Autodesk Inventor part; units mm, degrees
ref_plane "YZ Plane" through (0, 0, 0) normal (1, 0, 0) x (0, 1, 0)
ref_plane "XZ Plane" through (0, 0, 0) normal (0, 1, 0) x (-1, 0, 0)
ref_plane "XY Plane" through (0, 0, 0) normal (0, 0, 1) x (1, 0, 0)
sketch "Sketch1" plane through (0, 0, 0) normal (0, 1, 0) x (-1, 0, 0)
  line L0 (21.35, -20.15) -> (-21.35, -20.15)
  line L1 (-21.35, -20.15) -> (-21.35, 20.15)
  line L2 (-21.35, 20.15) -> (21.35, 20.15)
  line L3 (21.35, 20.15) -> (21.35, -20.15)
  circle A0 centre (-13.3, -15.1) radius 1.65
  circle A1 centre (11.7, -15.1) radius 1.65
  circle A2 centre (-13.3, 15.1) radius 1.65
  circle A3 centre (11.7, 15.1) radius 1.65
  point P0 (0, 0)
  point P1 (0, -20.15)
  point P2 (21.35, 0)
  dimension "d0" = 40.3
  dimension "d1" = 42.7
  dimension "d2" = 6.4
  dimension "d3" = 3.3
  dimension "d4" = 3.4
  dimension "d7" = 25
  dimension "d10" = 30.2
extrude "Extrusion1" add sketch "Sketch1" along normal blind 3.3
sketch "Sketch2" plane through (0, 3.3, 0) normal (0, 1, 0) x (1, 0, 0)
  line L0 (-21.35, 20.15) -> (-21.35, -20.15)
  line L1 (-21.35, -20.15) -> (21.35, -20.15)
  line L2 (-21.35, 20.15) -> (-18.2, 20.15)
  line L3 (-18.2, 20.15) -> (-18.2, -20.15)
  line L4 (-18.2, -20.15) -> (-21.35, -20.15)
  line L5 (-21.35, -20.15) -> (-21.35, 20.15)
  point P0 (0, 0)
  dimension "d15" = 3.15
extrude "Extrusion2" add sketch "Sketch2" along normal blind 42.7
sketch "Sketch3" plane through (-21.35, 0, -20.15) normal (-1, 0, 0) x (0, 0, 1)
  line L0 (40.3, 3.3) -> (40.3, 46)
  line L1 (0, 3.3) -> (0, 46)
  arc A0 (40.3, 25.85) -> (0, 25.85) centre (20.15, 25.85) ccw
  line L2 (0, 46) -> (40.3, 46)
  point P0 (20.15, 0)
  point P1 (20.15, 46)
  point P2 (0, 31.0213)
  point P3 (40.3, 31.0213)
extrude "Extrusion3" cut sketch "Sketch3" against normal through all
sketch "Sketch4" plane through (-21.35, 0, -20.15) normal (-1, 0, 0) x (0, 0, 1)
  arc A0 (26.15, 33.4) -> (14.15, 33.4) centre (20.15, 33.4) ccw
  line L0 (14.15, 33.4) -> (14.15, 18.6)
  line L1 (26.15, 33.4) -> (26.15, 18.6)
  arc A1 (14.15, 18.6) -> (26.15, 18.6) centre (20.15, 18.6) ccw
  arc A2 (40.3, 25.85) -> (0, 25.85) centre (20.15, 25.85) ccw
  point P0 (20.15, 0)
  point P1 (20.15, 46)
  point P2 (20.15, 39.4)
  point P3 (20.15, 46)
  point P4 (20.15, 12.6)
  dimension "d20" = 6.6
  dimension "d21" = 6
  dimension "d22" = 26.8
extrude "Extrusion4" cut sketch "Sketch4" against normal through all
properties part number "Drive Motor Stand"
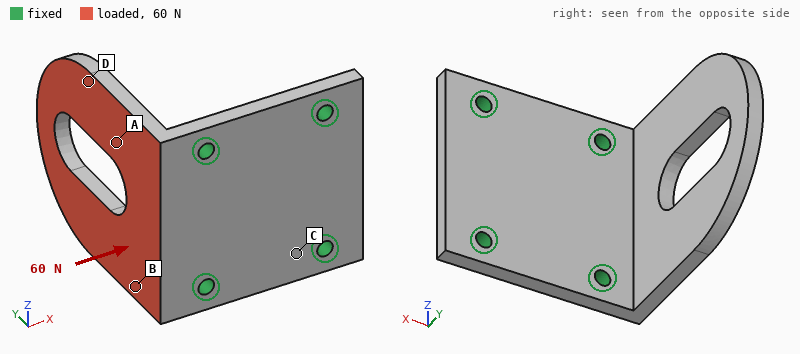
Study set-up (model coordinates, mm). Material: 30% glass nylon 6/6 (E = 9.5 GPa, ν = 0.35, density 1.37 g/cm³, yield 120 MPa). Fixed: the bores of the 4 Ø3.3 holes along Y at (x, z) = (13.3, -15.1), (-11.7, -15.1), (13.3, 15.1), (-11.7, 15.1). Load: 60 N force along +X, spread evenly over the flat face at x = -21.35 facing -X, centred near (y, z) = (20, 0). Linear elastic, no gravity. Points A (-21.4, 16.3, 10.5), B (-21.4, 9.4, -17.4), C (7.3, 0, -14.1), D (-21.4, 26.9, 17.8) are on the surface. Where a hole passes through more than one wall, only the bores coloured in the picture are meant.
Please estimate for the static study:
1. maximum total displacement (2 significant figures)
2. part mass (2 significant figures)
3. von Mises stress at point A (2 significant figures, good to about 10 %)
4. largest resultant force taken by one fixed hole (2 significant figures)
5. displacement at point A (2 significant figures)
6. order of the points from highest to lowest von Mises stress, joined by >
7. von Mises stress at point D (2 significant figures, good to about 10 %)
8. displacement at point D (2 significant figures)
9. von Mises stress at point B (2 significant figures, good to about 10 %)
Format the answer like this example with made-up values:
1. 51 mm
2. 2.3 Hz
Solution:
1. 0.87 mm
2. 13 g
3. 9.2 MPa
4. 23 N
5. 0.20 mm
6. B > A > D > C
7. 3.9 MPa
8. 0.41 mm
9. 12 MPa
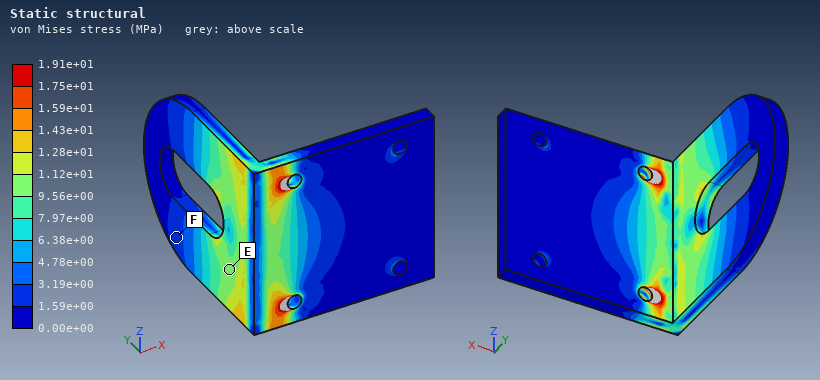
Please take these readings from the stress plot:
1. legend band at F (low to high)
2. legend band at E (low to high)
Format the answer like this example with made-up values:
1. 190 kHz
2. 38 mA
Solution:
1. 1.59e+00 to 3.19e+00 MPa
2. 9.56e+00 to 1.12e+01 MPa
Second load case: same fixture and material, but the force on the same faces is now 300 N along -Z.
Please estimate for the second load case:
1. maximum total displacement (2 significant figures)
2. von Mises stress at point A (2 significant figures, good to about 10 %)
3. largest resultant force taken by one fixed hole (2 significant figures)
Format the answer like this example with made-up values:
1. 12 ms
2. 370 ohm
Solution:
1. 0.20 mm
2. 7.1 MPa
3. 250 N
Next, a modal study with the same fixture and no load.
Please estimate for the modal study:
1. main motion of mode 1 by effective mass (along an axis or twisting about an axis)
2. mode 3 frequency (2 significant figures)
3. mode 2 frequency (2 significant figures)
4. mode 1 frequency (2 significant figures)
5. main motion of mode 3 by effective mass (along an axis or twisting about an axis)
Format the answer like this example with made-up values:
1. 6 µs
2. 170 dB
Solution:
1. along X
2. 2900 Hz
3. 1800 Hz
4. 690 Hz
5. along Z
